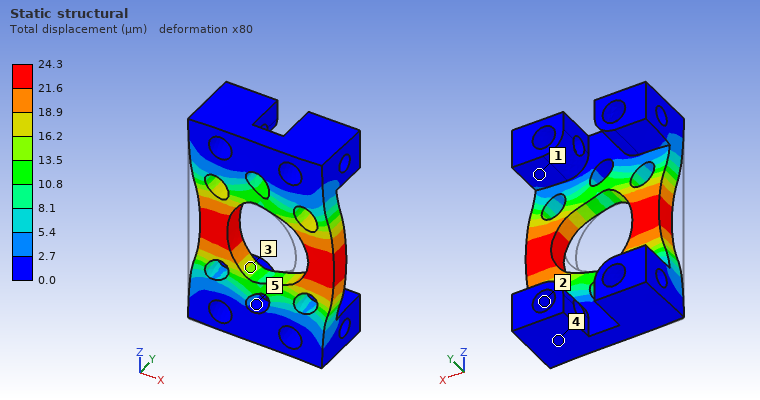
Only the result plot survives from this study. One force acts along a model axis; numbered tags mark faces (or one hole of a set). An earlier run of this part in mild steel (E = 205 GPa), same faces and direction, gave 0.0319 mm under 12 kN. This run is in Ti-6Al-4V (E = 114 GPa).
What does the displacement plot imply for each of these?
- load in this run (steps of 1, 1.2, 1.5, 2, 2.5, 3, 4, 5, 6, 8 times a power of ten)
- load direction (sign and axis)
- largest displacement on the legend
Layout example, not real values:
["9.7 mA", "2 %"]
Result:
["5 kN", "+X", "24.3 µm"]
